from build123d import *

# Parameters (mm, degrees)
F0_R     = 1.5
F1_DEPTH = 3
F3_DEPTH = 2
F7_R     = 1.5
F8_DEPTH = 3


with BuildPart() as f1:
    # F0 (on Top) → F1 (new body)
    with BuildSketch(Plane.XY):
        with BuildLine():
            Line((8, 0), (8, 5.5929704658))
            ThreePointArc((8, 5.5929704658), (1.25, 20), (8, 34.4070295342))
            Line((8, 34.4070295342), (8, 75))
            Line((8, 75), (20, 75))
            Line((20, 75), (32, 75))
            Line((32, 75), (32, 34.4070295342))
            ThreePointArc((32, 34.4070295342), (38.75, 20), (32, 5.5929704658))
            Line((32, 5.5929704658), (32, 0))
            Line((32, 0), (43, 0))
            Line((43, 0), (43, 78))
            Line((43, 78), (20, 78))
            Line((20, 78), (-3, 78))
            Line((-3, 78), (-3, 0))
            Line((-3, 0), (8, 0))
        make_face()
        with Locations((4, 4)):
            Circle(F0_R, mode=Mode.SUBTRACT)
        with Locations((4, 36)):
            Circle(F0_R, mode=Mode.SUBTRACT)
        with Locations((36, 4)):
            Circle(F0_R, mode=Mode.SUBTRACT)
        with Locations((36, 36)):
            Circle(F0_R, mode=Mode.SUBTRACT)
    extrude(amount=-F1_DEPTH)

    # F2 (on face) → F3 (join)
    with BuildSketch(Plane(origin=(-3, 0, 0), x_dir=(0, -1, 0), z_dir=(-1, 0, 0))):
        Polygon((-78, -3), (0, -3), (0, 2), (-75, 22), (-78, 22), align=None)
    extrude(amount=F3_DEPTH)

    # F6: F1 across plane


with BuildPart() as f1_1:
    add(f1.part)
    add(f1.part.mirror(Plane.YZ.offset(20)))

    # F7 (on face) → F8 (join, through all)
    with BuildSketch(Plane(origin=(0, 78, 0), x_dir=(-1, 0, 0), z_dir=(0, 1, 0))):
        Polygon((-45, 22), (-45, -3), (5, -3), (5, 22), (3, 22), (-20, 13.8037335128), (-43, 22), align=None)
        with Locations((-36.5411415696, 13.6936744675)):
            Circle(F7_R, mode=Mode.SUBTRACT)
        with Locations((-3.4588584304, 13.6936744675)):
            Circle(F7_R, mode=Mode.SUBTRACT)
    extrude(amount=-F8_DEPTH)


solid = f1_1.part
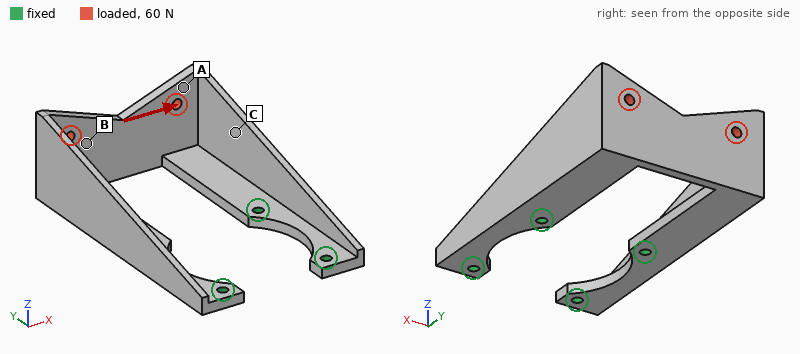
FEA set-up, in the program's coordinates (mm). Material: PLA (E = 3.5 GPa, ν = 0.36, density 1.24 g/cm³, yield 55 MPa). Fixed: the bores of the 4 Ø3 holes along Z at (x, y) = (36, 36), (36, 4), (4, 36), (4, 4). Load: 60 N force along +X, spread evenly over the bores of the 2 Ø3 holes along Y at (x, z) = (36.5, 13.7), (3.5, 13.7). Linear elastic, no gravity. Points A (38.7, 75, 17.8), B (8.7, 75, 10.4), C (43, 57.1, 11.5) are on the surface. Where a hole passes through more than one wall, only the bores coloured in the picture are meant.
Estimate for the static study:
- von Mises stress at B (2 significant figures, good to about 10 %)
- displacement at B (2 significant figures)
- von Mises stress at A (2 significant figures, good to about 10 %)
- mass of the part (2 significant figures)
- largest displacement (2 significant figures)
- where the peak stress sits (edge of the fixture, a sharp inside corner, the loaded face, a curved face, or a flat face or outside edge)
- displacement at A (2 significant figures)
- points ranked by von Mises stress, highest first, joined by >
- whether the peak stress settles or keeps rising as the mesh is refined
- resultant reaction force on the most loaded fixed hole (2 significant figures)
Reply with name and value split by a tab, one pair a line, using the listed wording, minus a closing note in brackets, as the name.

von Mises stress at B	5.6 MPa
displacement at B	0.66 mm
von Mises stress at A	4.1 MPa
mass of the part	15 g
largest displacement	1.0 mm
where the peak stress sits	edge of the fixture
displacement at A	0.86 mm
points ranked by von Mises stress, highest first, joined by >	B > A > C
whether the peak stress settles or keeps rising as the mesh is refined	keeps rising
resultant reaction force on the most loaded fixed hole	57 N
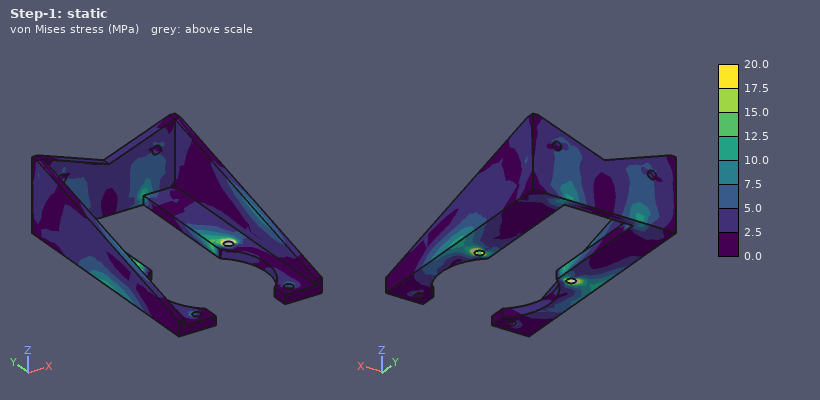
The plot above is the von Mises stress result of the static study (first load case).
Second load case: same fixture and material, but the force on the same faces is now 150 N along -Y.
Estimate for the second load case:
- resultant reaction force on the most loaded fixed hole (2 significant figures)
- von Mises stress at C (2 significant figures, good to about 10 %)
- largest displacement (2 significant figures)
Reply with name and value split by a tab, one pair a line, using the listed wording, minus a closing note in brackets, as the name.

resultant reaction force on the most loaded fixed hole	62 N
von Mises stress at C	4.8 MPa
largest displacement	0.75 mm
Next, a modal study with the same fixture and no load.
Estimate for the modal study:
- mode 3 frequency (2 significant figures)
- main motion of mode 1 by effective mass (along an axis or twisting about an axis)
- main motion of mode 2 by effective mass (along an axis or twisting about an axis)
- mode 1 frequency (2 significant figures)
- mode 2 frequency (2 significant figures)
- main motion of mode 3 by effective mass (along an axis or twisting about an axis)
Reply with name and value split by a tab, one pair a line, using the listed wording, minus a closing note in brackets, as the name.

mode 3 frequency	1100 Hz
main motion of mode 1 by effective mass	along X
main motion of mode 2 by effective mass	along Z
mode 1 frequency	590 Hz
mode 2 frequency	630 Hz
main motion of mode 3 by effective mass	along X
